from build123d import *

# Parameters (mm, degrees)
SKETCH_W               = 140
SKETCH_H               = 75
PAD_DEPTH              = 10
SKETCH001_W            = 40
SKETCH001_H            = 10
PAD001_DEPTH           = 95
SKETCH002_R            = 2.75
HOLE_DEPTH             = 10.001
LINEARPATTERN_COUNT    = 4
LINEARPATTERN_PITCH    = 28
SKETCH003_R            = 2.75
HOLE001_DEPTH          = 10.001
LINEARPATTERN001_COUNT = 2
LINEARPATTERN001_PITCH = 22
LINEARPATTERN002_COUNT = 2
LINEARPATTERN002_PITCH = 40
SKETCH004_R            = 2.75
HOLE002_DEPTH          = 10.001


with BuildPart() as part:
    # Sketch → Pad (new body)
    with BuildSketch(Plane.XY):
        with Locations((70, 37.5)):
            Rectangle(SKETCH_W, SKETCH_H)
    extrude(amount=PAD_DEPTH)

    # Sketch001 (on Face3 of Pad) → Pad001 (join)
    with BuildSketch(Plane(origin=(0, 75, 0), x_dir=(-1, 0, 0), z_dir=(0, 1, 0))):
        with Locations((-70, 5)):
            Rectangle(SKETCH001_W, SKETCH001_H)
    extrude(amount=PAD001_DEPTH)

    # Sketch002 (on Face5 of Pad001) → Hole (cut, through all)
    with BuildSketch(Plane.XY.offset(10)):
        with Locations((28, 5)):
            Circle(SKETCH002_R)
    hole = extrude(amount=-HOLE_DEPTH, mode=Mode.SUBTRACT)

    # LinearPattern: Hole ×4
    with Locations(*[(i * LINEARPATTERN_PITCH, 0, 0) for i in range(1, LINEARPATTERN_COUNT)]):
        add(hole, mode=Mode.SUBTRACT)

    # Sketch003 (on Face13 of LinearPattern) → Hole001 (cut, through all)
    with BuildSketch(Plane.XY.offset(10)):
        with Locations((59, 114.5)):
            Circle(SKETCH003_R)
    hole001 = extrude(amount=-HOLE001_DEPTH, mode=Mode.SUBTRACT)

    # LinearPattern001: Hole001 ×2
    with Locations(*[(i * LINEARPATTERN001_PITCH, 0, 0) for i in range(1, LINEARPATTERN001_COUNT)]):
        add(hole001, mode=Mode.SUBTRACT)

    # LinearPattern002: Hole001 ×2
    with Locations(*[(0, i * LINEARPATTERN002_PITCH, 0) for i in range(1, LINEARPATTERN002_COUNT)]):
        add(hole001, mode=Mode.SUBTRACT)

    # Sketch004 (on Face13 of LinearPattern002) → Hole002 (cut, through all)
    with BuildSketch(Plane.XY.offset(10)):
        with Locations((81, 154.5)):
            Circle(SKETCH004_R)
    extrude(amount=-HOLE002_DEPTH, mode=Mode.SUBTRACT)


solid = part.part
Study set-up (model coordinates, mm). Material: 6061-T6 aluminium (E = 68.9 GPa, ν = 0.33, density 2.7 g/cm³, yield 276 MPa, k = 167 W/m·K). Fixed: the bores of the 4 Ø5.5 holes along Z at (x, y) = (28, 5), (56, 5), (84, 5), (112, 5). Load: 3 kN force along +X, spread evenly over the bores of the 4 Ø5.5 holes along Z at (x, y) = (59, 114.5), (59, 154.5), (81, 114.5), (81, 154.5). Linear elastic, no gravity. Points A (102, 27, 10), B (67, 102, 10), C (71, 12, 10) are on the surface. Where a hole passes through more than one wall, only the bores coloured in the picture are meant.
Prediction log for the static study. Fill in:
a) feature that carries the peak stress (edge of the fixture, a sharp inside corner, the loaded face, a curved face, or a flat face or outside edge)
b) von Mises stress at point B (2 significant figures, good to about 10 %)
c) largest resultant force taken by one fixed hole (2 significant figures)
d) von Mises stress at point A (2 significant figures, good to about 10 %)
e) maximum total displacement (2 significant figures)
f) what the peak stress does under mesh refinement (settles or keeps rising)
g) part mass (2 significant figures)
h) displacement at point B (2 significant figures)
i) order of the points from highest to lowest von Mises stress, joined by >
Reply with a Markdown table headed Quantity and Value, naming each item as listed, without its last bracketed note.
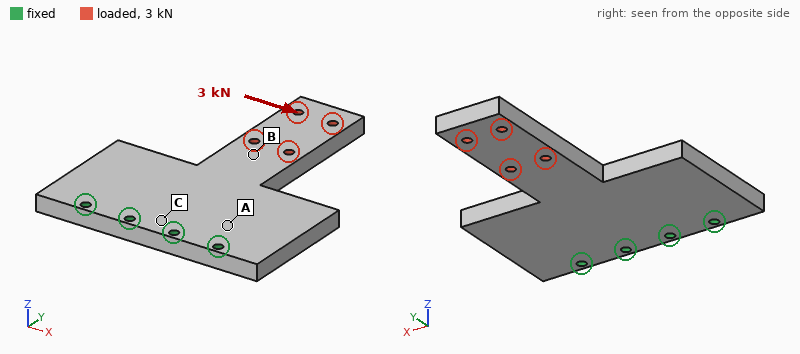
| Quantity | Value |
|---|---|
| feature that carries the peak stress | a sharp inside corner |
| von Mises stress at point B | 20 MPa |
| largest resultant force taken by one fixed hole | 4.1 kN |
| von Mises stress at point A | 15 MPa |
| maximum total displacement | 0.25 mm |
| what the peak stress does under mesh refinement | keeps rising |
| part mass | 380 g |
| displacement at point B | 0.069 mm |
| order of the points from highest to lowest von Mises stress, joined by > | B > A > C |
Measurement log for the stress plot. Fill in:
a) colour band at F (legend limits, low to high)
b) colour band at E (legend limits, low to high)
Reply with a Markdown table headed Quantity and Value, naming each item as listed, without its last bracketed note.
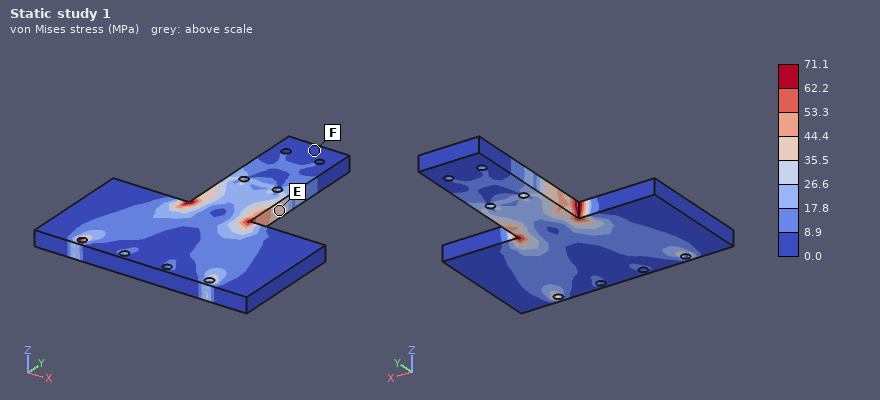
| Quantity | Value |
|---|---|
| colour band at F | 0.0 to 8.9 MPa |
| colour band at E | 35.5 to 44.4 MPa |
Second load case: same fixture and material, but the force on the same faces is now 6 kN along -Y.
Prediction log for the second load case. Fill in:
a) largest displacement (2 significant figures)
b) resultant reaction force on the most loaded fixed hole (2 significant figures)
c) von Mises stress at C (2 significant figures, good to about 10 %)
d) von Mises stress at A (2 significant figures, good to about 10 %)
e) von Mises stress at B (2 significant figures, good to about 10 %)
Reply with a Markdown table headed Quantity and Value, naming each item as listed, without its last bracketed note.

| Quantity | Value |
|---|---|
| largest displacement | 24 µm |
| resultant reaction force on the most loaded fixed hole | 1.6 kN |
| von Mises stress at C | 3.1 MPa |
| von Mises stress at A | 5.8 MPa |
| von Mises stress at B | 15 MPa |
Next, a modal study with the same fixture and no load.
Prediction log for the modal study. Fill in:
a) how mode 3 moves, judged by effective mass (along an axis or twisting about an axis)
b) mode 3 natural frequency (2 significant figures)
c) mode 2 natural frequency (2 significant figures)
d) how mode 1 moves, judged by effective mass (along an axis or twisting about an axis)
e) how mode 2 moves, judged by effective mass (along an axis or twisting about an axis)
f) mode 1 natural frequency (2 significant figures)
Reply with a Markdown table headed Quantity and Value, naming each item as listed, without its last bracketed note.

| Quantity | Value |
|---|---|
| how mode 3 moves, judged by effective mass | twisting about Y |
| mode 3 natural frequency | 2000 Hz |
| mode 2 natural frequency | 1700 Hz |
| how mode 1 moves, judged by effective mass | along Z |
| how mode 2 moves, judged by effective mass | along Z |
| mode 1 natural frequency | 440 Hz |
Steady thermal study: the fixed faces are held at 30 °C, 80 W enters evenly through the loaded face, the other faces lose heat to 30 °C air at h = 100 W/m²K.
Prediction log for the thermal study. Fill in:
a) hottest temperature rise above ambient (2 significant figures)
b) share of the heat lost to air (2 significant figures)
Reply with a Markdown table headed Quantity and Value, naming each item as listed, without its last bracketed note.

| Quantity | Value |
|---|---|
| hottest temperature rise above ambient | 57 K |
| share of the heat lost to air | 65 % |
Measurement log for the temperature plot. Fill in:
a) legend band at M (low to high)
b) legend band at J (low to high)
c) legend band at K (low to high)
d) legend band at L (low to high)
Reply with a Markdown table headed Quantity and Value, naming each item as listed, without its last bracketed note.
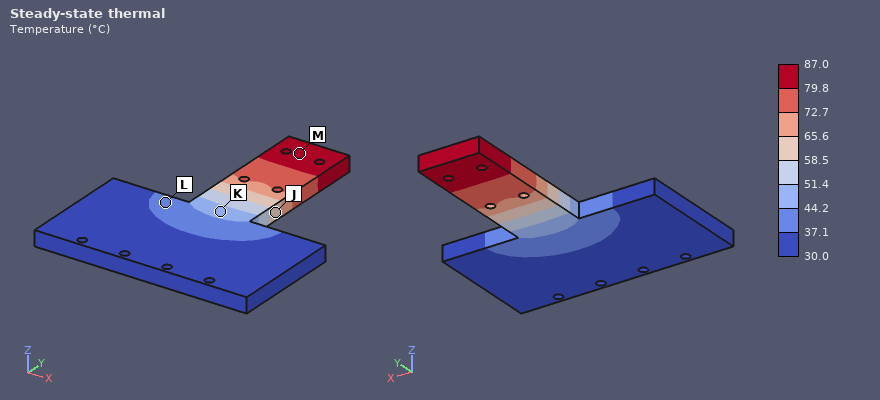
| Quantity | Value |
|---|---|
| legend band at M | 79.8 to 87.0 °C |
| legend band at J | 58.5 to 65.6 °C |
| legend band at K | 44.2 to 51.4 °C |
| legend band at L | 37.1 to 44.2 °C |
